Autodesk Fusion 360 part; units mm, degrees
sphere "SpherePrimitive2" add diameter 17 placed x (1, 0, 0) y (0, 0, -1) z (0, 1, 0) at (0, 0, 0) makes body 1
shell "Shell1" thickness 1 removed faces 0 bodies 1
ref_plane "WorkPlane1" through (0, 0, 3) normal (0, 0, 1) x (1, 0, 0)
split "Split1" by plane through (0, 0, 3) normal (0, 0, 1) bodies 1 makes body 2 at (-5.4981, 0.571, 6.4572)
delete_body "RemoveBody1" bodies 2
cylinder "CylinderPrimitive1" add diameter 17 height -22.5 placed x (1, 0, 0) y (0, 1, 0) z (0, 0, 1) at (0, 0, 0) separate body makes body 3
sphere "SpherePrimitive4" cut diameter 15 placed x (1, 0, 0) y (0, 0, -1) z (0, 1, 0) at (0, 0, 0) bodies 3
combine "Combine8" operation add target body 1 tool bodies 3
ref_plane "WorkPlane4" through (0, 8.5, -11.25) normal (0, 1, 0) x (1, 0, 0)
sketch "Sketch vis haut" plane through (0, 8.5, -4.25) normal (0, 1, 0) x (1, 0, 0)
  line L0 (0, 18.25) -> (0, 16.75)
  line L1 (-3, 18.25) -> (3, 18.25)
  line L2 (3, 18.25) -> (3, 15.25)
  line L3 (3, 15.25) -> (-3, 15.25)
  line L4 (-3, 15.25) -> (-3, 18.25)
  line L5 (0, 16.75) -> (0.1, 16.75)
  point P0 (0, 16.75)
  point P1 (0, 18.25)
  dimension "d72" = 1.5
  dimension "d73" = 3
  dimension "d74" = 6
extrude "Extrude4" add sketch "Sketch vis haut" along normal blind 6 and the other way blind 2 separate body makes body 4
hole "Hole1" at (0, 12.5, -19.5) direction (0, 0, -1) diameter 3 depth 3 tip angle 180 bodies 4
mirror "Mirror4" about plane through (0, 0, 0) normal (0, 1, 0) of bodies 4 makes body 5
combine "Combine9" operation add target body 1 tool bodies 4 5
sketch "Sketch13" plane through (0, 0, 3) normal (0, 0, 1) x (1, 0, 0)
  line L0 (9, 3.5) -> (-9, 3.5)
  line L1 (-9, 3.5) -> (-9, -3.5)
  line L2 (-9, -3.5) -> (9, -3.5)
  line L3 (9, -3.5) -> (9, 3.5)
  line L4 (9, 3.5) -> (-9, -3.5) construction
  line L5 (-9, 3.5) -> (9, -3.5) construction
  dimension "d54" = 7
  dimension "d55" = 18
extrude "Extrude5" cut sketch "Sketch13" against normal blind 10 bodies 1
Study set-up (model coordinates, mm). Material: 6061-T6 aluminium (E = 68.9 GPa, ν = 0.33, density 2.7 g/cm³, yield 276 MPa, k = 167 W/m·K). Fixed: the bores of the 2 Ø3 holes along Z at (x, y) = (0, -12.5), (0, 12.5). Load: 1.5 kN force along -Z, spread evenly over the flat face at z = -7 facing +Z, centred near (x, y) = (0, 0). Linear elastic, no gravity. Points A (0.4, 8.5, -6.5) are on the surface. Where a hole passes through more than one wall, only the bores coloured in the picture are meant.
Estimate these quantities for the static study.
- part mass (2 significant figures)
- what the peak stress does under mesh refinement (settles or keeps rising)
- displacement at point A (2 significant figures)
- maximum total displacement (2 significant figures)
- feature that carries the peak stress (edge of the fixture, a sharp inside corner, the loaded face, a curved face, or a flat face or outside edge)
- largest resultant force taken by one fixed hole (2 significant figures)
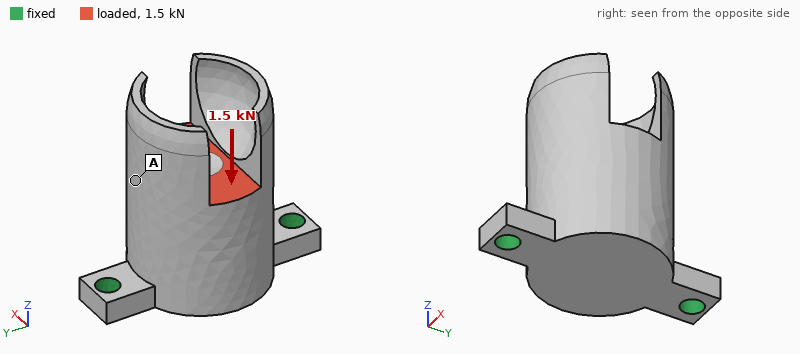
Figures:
12 g
keeps rising
15 µm
18 µm
edge of the fixture
830 N
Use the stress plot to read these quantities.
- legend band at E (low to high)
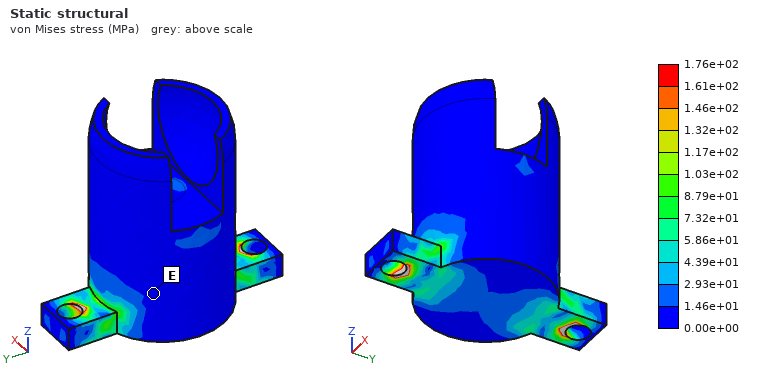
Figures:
0.00e+00 to 1.46e+01 MPa
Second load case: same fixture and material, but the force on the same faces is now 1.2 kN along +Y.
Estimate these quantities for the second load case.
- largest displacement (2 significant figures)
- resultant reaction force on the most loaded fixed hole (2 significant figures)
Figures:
50 µm
1.0 kN
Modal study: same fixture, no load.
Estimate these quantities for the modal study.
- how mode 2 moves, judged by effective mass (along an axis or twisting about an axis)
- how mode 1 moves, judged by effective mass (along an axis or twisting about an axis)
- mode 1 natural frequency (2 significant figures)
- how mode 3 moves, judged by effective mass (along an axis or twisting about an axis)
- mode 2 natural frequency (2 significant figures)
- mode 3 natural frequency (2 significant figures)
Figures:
along Y
along X
3200 Hz
along Z
13 kHz
15 kHz
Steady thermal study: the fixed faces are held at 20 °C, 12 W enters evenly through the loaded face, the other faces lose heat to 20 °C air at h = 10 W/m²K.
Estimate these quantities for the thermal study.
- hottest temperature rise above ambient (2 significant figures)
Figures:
15 K
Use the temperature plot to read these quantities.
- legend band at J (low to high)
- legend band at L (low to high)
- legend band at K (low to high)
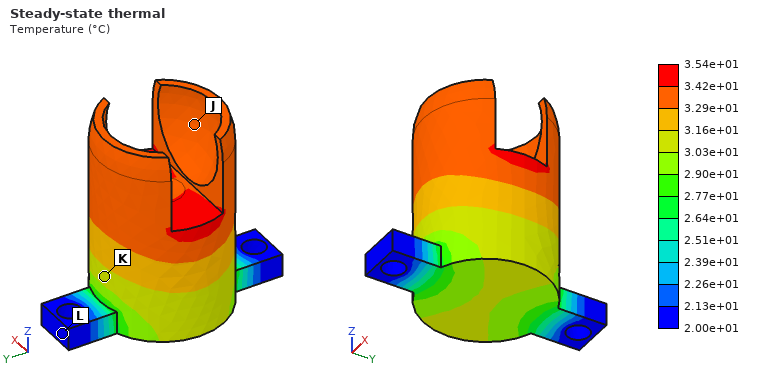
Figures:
3.29e+01 to 3.42e+01 °C
2.00e+01 to 2.13e+01 °C
3.03e+01 to 3.16e+01 °C
